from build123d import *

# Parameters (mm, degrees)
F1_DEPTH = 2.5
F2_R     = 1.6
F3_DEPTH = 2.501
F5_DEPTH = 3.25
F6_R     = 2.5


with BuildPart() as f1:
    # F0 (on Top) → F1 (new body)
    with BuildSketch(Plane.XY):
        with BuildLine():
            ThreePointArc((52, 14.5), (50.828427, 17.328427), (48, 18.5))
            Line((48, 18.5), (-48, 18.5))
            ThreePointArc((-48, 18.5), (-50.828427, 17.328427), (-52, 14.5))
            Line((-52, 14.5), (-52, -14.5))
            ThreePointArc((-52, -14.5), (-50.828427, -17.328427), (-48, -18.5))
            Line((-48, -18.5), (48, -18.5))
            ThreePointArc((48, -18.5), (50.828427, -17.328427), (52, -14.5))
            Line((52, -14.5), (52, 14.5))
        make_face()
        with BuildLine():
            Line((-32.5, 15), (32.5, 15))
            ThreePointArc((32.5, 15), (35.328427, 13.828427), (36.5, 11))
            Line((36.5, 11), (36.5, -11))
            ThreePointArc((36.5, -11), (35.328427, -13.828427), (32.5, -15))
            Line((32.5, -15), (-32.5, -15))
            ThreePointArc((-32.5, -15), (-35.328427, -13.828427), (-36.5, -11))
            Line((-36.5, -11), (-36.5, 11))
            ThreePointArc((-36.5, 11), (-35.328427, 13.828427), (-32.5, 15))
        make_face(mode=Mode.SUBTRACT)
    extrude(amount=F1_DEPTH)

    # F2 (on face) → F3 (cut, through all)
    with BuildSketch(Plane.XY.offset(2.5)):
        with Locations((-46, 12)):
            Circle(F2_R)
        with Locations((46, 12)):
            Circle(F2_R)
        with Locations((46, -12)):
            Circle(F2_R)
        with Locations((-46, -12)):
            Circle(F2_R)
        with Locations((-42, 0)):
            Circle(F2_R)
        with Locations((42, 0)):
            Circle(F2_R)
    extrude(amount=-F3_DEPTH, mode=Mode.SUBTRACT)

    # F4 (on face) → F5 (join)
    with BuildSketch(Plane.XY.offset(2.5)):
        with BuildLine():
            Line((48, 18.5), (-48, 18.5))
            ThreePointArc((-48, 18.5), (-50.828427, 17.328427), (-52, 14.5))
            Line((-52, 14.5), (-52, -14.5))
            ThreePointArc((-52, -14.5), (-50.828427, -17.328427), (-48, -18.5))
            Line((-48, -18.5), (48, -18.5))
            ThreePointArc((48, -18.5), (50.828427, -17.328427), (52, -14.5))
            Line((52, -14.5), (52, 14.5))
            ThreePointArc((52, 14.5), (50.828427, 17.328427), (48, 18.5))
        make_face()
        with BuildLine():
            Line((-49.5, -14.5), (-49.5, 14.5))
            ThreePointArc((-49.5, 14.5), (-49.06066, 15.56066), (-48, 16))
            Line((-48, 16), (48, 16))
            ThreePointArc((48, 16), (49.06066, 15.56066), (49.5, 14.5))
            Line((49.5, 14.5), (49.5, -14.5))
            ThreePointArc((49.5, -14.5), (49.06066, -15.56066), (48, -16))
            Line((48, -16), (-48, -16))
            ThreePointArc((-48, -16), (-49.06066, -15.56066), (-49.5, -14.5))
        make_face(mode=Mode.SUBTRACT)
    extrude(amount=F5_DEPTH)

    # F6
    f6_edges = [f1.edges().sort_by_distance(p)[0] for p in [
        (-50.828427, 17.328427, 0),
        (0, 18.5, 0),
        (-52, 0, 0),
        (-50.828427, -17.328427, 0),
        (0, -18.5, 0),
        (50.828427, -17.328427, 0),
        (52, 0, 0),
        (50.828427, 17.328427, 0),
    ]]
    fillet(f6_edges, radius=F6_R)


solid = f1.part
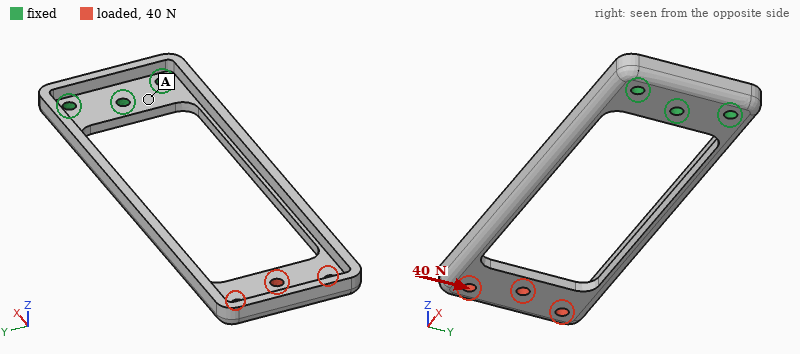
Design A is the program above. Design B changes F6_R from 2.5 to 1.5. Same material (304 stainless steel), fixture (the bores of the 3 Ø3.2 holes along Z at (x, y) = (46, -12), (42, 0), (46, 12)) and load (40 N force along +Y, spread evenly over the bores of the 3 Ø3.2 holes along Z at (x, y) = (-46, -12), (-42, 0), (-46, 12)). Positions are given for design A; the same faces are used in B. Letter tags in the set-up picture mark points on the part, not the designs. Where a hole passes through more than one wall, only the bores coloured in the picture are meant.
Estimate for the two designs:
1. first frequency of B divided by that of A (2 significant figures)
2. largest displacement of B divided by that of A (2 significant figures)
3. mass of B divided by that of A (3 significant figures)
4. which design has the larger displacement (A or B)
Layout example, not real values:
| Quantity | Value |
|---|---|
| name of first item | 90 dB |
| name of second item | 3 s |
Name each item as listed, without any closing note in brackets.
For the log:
| Quantity | Value |
|---|---|
| first frequency of B divided by that of A | 1.0 |
| largest displacement of B divided by that of A | 0.89 |
| mass of B divided by that of A | 1.04 |
| which design has the larger displacement | A |
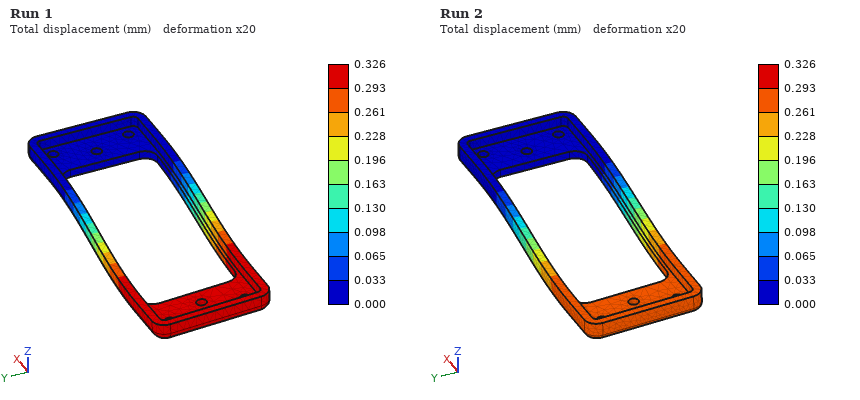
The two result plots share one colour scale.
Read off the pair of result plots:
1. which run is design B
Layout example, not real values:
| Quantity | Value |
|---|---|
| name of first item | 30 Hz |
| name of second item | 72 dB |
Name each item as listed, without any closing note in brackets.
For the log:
| Quantity | Value |
|---|---|
| which run is design B | Run 2 |
